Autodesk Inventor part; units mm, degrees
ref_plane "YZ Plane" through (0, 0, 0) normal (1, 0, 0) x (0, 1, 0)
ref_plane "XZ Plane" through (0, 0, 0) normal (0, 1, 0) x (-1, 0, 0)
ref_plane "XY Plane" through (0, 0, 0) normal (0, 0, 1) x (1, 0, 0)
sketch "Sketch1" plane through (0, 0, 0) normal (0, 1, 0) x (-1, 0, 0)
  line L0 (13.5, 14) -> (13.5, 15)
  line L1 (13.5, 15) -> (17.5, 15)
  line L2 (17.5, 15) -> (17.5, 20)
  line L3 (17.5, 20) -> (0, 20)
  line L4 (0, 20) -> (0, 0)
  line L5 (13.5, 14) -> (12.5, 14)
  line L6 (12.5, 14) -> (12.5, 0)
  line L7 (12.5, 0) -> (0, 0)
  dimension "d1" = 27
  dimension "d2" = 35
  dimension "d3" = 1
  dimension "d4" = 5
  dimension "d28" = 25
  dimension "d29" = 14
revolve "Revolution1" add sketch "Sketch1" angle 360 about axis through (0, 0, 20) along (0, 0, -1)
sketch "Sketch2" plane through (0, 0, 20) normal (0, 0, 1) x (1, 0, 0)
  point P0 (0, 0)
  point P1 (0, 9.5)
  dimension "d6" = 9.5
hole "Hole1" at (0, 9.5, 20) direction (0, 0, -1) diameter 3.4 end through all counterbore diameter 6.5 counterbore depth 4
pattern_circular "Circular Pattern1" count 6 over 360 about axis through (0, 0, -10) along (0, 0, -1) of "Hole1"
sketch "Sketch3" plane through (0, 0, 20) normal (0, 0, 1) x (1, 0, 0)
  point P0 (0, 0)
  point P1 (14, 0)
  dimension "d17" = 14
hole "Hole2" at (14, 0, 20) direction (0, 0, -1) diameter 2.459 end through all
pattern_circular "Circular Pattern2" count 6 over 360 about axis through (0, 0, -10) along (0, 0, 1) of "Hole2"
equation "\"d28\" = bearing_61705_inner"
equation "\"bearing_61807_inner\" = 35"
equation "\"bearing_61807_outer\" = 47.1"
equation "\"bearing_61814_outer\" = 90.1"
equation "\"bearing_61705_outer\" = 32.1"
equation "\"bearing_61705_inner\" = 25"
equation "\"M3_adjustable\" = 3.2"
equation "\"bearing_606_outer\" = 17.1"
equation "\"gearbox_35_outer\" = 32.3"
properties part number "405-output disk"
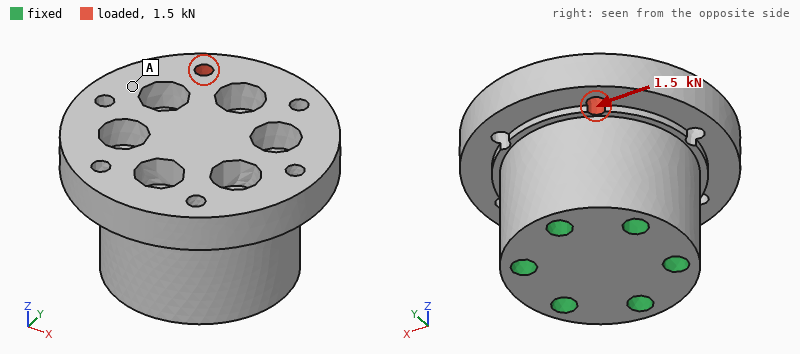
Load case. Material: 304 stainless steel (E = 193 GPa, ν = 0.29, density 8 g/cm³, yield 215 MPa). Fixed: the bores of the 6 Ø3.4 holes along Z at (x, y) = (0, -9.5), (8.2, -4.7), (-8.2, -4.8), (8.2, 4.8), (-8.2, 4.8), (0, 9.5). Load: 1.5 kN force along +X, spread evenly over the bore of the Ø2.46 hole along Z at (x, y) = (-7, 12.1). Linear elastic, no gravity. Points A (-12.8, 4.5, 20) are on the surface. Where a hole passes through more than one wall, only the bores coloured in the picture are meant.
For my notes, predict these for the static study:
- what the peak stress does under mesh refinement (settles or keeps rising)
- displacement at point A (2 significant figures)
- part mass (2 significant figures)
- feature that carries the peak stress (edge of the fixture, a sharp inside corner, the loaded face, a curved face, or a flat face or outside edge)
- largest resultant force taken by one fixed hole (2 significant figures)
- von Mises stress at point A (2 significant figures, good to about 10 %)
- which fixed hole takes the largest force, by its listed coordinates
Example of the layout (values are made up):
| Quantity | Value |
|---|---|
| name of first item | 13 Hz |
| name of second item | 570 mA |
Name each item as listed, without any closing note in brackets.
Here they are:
| Quantity | Value |
|---|---|
| what the peak stress does under mesh refinement | keeps rising |
| displacement at point A | 0.94 µm |
| part mass | 84 g |
| feature that carries the peak stress | edge of the fixture |
| largest resultant force taken by one fixed hole | 860 N |
| von Mises stress at point A | 8.1 MPa |
| which fixed hole takes the largest force, by its listed coordinates | (0, 9.5) |
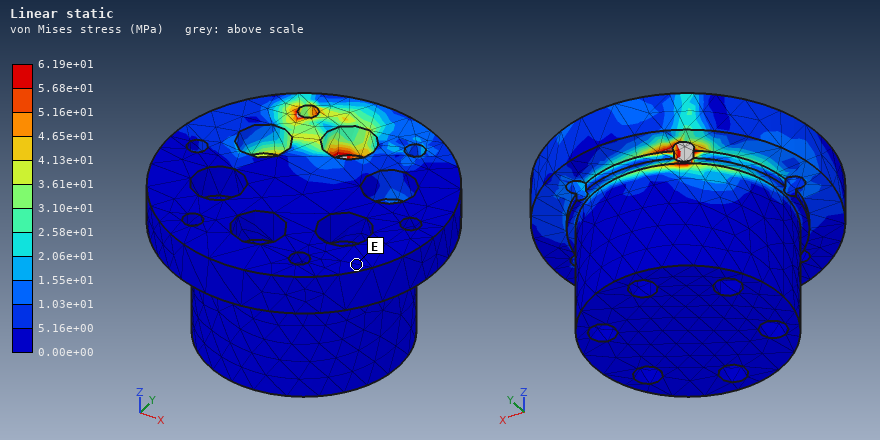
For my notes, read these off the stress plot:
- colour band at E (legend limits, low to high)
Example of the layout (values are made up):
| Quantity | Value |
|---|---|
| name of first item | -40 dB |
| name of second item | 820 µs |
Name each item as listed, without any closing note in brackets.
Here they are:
| Quantity | Value |
|---|---|
| colour band at E | 0.00e+00 to 5.16e+00 MPa |
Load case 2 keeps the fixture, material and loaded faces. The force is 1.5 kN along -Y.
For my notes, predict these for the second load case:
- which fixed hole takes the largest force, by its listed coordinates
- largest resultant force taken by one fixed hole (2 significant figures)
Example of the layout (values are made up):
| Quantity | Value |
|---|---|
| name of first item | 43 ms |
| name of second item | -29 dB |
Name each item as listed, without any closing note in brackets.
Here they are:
| Quantity | Value |
|---|---|
| which fixed hole takes the largest force, by its listed coordinates | (-8.2, 4.8) |
| largest resultant force taken by one fixed hole | 760 N |
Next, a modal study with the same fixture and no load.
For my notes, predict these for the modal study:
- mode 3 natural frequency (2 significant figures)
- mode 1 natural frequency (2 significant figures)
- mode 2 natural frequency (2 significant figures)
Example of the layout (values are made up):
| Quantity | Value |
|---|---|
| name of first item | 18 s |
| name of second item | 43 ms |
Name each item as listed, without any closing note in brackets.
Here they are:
| Quantity | Value |
|---|---|
| mode 3 natural frequency | 45 kHz |
| mode 1 natural frequency | 42 kHz |
| mode 2 natural frequency | 42 kHz |
